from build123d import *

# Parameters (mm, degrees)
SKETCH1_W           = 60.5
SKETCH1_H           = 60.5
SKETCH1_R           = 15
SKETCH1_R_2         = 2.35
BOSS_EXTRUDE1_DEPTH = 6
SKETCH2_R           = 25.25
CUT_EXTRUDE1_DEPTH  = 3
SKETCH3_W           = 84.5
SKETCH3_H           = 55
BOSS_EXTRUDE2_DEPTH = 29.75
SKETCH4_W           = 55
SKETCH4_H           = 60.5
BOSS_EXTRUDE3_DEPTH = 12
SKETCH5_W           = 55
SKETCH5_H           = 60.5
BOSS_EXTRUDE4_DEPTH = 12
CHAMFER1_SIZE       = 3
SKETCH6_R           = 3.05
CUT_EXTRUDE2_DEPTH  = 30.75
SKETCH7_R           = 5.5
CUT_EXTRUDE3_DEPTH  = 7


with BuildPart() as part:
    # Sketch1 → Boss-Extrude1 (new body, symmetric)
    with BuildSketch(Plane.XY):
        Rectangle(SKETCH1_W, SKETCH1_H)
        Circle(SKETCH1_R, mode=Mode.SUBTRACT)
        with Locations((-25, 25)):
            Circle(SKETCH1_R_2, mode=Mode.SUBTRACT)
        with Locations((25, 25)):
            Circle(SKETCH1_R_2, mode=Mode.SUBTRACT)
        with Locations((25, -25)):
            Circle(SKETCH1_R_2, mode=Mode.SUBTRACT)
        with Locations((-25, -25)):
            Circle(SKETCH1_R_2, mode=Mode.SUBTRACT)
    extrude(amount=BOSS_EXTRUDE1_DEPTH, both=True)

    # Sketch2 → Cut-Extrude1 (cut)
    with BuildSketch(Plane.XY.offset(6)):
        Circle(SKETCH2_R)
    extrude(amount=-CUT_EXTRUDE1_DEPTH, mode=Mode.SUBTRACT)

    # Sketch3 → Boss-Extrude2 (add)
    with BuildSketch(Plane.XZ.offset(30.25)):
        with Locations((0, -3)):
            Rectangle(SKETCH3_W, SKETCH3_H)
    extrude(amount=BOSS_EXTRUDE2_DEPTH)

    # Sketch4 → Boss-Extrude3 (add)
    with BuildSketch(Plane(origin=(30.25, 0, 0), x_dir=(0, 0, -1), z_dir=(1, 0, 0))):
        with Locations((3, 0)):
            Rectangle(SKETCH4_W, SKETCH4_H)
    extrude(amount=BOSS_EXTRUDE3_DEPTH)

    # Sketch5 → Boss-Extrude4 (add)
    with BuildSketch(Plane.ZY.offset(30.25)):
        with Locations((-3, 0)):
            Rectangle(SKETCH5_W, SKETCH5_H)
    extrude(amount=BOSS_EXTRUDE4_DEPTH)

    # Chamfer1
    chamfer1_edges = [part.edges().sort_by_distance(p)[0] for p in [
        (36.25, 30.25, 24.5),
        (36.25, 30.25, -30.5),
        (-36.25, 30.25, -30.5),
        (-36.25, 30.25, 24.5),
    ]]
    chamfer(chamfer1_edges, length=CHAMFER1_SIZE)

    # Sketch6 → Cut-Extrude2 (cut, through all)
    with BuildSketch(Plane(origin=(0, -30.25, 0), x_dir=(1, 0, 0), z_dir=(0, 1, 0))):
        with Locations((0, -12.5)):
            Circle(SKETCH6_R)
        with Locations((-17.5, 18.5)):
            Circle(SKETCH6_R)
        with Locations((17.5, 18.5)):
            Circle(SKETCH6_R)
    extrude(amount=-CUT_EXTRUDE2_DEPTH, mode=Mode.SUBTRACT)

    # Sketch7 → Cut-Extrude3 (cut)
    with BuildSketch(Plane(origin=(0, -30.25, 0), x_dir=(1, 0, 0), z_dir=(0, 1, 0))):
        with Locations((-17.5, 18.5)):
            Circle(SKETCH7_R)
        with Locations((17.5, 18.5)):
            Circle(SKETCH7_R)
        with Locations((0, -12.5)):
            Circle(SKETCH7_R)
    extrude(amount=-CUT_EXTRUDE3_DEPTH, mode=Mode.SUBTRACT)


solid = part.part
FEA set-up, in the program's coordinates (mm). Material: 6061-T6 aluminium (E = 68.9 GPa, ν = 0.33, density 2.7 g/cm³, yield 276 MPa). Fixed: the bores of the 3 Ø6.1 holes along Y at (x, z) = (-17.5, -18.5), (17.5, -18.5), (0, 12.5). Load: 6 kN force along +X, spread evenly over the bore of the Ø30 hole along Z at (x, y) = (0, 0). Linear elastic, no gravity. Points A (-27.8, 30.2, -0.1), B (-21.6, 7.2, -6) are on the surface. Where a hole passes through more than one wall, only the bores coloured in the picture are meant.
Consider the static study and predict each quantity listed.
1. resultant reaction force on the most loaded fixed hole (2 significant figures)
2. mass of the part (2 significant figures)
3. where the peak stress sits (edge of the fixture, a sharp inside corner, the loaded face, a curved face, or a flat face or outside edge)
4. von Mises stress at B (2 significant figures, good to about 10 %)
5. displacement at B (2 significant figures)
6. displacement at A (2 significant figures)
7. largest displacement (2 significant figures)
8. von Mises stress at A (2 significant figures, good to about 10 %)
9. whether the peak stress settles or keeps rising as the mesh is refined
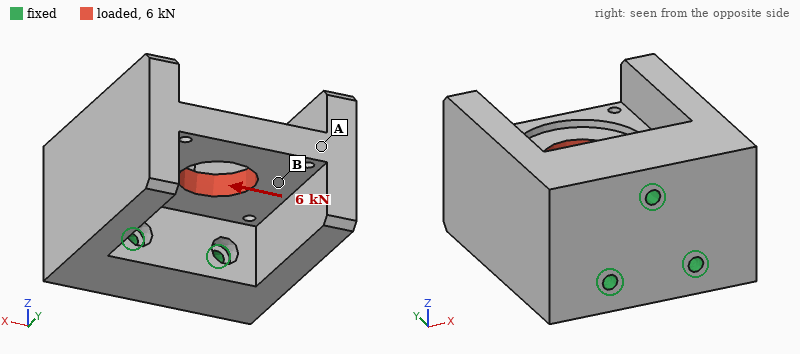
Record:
4.5 kN
660 g
edge of the fixture
15 MPa
33 µm
43 µm
48 µm
5.0 MPa
keeps rising
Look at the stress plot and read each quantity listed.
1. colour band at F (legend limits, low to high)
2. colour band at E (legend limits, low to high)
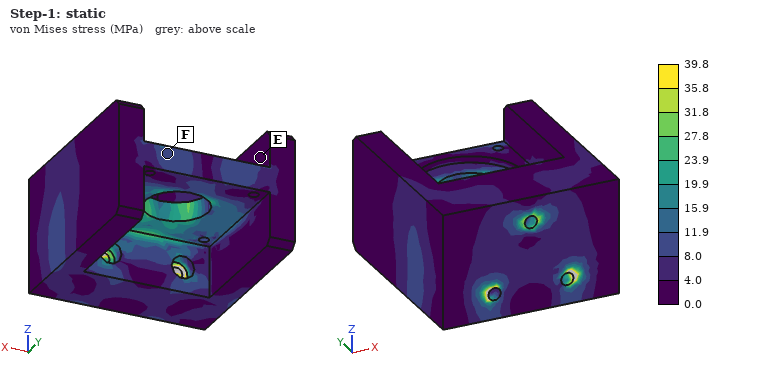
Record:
8.0 to 11.9 MPa
0.0 to 4.0 MPa
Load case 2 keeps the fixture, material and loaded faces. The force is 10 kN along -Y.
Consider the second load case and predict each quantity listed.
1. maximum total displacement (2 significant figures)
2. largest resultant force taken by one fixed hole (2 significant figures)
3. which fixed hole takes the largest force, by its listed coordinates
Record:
22 µm
4.4 kN
(0, 12.5)
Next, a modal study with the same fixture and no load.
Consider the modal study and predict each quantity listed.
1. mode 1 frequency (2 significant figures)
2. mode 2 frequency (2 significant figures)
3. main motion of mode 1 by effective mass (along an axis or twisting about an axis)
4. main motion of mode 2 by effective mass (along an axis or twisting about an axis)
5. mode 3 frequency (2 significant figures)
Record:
3500 Hz
3800 Hz
along X
along Z
4800 Hz
